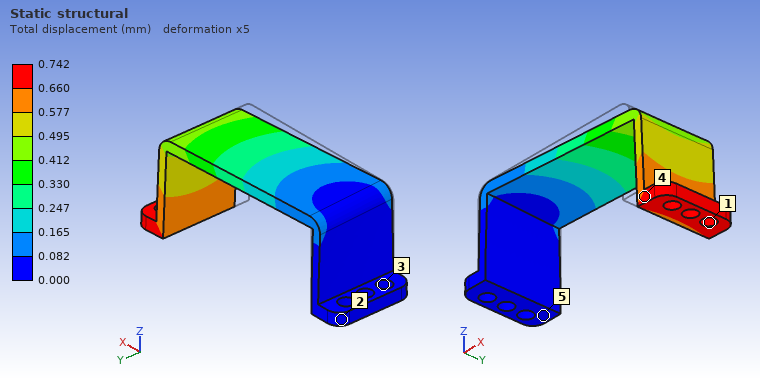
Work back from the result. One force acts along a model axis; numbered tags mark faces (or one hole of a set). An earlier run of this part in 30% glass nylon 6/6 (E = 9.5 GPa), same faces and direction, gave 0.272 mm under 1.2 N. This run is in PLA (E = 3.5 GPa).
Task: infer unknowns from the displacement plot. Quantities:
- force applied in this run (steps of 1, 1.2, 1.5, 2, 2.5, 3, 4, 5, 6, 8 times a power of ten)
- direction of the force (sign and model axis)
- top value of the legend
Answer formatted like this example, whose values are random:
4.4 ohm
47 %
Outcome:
1.2 N
+Y
0.742 mm
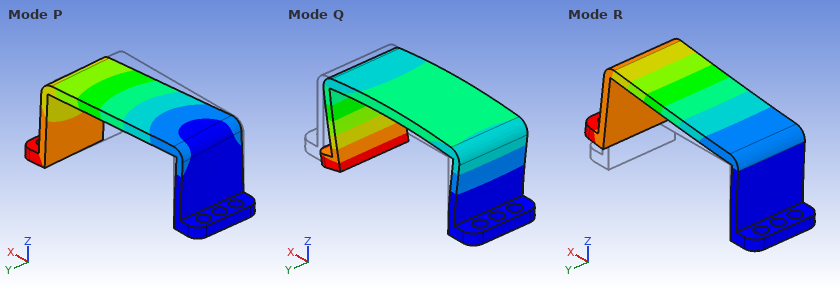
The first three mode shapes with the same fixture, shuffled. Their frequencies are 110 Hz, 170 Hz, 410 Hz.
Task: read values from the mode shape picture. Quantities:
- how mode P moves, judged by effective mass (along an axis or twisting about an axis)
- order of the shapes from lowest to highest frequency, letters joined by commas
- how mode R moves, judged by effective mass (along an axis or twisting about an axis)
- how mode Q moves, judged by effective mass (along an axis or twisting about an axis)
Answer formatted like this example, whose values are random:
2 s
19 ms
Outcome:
along Y
R, P, Q
along Z
along X
